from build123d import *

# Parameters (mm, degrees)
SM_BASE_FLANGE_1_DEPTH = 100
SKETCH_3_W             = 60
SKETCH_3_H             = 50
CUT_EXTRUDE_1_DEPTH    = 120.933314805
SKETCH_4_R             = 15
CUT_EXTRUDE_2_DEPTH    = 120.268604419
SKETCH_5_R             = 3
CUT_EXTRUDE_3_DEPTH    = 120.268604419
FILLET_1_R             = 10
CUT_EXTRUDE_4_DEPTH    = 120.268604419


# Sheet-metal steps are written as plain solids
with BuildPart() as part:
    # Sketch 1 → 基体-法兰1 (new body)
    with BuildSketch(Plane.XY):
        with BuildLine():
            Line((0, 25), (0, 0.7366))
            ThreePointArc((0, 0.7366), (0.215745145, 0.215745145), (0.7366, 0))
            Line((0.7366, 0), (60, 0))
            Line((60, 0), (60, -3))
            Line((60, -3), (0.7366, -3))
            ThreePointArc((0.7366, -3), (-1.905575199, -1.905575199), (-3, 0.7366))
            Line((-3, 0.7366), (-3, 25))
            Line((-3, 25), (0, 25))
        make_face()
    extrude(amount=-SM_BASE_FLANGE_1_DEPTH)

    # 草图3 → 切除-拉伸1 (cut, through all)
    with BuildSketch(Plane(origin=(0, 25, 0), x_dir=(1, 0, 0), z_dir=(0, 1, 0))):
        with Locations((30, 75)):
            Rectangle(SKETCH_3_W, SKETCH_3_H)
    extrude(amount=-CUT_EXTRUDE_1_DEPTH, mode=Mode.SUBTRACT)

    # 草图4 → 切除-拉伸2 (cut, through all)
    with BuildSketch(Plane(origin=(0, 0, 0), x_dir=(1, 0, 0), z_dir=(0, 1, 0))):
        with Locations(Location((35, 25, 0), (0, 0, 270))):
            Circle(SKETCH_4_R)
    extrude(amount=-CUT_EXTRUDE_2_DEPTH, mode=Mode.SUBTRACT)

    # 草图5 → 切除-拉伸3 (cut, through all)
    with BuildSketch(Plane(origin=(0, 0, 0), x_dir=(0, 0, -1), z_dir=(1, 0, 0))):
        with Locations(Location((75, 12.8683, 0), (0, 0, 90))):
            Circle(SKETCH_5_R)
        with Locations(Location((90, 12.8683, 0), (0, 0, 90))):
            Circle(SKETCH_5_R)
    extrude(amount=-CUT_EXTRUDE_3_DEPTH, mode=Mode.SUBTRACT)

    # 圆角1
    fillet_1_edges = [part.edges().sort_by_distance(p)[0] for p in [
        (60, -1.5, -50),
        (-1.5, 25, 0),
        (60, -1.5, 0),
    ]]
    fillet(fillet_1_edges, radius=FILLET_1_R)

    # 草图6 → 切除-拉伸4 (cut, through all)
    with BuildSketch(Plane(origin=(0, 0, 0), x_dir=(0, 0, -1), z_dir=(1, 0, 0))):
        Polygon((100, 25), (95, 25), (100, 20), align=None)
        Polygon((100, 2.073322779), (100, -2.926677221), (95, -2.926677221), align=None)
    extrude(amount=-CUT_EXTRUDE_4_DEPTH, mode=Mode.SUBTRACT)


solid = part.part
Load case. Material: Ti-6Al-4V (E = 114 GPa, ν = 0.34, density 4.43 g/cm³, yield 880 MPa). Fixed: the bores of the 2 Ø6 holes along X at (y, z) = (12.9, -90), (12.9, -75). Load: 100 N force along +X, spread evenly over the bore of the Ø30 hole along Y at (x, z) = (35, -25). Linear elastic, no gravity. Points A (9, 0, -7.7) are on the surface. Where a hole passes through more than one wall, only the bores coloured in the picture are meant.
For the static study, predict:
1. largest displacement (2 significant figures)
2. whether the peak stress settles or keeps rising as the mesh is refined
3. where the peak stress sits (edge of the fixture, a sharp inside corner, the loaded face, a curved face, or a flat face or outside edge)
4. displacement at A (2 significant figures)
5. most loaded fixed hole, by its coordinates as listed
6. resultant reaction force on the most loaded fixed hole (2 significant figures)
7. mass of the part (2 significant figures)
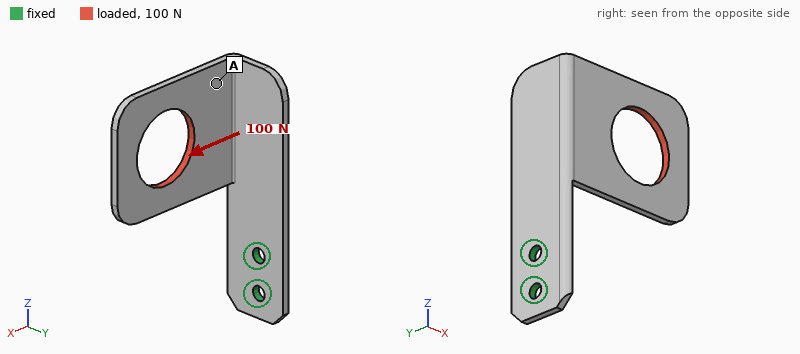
1.4 mm
keeps rising
a sharp inside corner
0.89 mm
(12.9, -75)
170 N
65 g
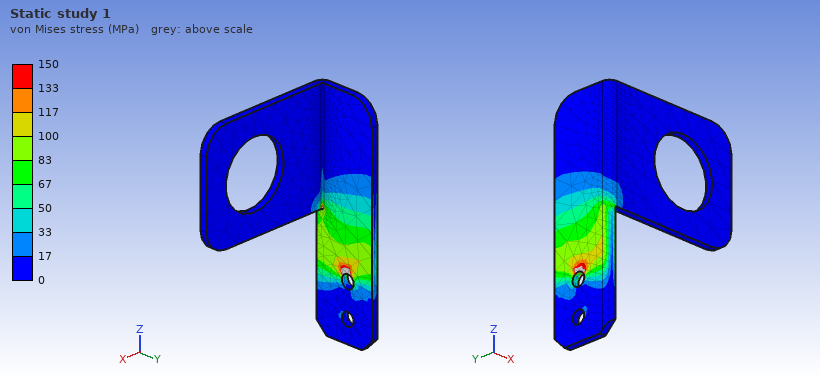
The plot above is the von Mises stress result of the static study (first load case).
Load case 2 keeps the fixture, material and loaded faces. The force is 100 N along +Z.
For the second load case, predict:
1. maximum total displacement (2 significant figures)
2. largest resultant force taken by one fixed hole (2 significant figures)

1.4 mm
97 N
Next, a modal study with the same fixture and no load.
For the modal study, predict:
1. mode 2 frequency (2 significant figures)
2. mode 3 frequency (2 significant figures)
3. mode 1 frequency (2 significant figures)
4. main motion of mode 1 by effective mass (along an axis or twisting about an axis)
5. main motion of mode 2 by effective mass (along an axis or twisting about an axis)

360 Hz
1400 Hz
230 Hz
along X
along Y
